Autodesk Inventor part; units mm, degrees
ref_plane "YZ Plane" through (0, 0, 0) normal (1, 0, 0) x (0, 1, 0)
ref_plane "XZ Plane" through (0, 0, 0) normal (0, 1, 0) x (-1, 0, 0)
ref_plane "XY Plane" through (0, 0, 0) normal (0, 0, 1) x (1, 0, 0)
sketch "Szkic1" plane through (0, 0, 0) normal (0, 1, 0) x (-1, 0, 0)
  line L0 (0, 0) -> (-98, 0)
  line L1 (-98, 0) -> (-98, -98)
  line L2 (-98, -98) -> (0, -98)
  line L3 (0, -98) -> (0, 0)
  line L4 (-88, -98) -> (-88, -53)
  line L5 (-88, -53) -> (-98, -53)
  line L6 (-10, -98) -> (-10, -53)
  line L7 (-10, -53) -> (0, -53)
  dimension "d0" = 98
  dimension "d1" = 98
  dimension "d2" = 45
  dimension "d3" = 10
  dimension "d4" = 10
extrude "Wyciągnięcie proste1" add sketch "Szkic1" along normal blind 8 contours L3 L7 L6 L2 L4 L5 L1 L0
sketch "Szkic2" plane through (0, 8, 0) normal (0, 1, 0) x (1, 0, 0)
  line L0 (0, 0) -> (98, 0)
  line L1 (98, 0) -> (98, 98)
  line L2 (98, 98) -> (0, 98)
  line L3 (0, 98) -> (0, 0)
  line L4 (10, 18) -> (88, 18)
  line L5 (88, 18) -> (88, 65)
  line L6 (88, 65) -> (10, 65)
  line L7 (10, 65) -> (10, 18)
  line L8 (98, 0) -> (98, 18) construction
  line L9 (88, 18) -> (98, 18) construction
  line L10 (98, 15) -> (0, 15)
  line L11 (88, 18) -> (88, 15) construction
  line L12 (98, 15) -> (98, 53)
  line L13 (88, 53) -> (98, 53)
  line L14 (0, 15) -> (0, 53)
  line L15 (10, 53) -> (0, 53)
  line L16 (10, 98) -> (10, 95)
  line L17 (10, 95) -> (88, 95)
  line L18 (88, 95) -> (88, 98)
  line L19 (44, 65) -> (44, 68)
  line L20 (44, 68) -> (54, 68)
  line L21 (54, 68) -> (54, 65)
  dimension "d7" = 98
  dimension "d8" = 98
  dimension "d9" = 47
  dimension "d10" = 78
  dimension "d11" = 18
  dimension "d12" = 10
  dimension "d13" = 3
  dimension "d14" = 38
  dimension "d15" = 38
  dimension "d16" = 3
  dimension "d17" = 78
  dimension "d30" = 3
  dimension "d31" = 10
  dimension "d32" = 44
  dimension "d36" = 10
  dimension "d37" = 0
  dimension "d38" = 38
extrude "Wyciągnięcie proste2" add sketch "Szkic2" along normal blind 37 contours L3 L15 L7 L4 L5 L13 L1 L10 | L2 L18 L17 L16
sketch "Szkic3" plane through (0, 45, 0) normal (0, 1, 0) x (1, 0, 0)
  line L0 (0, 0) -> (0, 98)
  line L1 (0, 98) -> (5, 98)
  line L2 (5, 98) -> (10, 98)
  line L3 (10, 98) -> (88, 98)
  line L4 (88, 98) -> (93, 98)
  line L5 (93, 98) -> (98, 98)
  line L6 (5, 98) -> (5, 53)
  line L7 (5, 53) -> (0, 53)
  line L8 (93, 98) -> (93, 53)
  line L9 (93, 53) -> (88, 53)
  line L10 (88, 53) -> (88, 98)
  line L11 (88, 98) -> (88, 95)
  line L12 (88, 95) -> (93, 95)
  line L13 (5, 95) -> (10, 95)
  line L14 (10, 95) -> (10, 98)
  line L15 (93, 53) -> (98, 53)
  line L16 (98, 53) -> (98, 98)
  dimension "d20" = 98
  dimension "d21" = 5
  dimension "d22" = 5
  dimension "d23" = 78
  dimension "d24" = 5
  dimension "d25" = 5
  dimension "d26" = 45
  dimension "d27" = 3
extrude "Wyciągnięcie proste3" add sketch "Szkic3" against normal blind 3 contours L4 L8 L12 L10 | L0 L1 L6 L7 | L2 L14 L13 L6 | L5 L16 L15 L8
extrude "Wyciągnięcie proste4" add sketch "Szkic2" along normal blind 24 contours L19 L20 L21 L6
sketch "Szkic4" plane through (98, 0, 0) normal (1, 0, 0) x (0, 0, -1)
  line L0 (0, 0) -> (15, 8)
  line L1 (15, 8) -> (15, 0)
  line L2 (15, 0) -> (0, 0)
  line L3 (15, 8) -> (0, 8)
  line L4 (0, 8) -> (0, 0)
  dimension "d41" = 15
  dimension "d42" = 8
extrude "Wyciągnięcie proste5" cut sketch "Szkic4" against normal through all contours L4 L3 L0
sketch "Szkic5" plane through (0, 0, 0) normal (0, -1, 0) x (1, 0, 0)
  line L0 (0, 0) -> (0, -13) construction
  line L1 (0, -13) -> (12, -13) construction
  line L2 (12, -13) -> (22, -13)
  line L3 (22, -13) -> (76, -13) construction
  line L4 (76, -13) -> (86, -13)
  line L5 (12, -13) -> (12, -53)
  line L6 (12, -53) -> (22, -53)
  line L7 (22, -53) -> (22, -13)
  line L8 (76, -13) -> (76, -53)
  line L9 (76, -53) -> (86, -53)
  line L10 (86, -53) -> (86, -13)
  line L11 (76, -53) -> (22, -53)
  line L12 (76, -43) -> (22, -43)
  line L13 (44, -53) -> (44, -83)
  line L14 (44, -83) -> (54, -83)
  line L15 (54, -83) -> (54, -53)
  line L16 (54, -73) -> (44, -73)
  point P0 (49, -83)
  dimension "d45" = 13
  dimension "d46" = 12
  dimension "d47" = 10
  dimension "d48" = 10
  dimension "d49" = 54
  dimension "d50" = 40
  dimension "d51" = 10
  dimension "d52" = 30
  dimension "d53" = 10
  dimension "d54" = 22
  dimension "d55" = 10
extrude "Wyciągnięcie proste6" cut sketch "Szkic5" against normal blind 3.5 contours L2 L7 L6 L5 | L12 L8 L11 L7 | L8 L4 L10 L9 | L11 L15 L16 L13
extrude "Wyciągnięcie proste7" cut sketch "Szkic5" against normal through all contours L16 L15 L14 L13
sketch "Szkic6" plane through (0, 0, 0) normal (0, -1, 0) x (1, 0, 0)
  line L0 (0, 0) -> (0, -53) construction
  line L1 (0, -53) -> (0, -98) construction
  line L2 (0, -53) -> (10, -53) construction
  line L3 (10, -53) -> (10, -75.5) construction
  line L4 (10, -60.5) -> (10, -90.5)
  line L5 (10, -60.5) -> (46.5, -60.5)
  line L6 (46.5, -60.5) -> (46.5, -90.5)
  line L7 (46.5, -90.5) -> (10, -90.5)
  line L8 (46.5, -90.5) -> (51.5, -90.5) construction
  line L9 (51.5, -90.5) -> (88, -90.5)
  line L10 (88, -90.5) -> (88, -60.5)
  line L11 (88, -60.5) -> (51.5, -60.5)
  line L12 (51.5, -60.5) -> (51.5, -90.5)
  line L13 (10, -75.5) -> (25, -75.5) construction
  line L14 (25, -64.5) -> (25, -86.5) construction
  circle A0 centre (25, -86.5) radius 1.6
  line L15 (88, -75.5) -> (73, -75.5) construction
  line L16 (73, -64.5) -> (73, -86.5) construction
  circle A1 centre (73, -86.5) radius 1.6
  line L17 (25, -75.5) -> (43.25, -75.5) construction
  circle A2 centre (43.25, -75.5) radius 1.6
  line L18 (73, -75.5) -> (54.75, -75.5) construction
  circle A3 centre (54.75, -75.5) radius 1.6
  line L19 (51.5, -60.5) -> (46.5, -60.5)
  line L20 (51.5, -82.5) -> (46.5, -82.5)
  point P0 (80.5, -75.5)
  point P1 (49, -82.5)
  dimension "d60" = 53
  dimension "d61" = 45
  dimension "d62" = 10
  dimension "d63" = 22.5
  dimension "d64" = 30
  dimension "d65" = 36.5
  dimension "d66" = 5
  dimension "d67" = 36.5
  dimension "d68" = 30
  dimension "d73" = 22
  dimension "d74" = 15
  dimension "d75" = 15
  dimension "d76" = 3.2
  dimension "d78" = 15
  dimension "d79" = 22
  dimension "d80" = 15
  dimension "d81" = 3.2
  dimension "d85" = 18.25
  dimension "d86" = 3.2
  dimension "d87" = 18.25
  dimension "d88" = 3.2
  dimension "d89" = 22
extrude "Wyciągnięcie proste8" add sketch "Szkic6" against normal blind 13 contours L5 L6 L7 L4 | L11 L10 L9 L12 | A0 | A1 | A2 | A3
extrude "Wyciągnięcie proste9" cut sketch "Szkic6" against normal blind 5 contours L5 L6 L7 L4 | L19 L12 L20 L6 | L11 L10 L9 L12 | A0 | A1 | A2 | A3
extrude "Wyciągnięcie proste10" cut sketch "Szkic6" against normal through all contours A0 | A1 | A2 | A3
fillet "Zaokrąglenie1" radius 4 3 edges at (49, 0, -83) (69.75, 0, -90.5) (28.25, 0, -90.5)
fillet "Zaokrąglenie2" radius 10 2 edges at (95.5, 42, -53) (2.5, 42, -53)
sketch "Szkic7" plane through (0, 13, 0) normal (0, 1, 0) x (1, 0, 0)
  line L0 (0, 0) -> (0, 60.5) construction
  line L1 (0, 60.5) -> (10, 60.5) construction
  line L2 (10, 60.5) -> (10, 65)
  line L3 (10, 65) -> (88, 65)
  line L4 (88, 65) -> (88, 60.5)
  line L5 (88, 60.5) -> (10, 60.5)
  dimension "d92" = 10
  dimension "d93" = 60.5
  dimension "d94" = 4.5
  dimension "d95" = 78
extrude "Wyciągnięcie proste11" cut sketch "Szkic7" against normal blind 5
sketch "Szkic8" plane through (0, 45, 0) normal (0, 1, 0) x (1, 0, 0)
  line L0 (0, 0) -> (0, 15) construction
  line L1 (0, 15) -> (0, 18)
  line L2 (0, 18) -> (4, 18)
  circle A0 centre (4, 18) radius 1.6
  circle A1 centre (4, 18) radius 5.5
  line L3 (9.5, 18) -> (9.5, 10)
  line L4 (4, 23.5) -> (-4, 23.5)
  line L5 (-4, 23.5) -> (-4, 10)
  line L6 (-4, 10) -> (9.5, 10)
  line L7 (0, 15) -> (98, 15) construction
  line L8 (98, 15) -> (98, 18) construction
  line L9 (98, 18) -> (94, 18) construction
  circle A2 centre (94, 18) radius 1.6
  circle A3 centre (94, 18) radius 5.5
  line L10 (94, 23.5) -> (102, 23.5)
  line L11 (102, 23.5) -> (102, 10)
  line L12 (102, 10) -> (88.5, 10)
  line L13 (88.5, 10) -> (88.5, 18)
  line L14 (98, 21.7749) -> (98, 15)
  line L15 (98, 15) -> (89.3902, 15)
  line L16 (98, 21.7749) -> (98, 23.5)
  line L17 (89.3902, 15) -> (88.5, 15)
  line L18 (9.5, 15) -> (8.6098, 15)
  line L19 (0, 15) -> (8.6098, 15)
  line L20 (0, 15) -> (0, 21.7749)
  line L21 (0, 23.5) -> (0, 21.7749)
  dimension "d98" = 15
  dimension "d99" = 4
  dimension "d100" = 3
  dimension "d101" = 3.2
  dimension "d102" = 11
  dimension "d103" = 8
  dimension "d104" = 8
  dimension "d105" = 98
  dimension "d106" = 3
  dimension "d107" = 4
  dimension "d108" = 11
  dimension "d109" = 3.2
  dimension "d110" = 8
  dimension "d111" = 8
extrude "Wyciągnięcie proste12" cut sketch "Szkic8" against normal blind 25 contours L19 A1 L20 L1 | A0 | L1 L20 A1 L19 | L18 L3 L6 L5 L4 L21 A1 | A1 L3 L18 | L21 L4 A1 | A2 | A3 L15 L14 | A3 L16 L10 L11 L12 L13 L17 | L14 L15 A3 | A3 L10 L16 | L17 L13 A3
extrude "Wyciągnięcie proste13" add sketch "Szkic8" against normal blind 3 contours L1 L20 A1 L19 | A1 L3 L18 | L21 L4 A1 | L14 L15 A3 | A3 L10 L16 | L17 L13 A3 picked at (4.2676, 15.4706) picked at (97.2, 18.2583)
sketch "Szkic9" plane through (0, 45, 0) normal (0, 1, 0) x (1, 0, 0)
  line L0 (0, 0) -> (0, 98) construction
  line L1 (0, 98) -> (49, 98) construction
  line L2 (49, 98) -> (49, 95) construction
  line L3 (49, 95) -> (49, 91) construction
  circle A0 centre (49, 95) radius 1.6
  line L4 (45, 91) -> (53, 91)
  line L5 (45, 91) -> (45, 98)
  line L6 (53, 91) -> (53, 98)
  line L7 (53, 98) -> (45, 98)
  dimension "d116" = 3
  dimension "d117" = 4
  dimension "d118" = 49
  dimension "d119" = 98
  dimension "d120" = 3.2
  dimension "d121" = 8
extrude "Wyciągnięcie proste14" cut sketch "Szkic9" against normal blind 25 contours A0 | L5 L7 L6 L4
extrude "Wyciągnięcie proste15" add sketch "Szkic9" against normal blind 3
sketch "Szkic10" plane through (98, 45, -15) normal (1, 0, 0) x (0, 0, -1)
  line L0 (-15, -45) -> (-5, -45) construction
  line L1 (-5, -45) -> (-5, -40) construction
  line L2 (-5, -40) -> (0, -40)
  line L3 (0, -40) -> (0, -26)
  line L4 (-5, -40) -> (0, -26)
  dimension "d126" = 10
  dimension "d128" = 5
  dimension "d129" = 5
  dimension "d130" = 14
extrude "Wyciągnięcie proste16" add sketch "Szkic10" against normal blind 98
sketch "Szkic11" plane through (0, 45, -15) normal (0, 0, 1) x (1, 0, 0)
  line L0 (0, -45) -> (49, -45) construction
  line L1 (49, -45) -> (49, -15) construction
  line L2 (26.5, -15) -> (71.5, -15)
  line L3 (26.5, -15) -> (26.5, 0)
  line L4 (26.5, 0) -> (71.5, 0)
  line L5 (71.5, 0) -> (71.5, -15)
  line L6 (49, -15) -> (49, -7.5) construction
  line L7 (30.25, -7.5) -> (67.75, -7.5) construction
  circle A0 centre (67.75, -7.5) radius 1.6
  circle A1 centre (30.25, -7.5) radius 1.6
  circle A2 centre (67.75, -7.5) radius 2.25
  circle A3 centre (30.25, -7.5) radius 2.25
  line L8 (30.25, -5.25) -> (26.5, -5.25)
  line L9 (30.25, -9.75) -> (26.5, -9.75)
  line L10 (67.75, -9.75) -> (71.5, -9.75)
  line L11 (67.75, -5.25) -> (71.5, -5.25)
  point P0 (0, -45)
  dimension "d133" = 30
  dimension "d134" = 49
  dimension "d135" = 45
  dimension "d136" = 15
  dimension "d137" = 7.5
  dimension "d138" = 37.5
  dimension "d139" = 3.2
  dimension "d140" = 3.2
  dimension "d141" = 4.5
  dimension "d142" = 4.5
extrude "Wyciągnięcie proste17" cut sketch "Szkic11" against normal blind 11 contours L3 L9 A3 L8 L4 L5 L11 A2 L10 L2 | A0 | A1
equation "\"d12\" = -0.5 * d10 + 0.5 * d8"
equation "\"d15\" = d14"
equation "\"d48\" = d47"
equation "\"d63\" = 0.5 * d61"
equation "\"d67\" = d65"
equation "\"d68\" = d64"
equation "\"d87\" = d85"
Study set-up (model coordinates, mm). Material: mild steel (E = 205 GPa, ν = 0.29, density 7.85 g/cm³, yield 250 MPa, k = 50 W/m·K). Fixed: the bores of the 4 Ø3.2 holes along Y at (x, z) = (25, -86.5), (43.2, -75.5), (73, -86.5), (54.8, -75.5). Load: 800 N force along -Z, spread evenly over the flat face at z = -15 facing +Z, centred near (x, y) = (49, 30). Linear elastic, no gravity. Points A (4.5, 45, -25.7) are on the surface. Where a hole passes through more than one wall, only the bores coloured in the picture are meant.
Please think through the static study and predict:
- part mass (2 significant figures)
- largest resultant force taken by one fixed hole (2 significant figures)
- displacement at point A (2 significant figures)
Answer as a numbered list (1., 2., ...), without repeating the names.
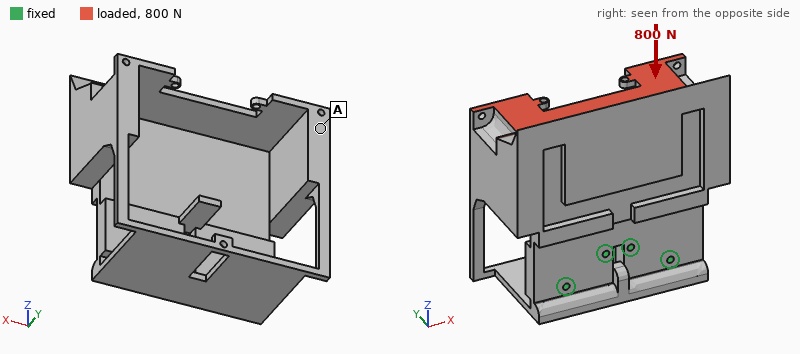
1. 790 g
2. 350 N
3. 0.16 mm
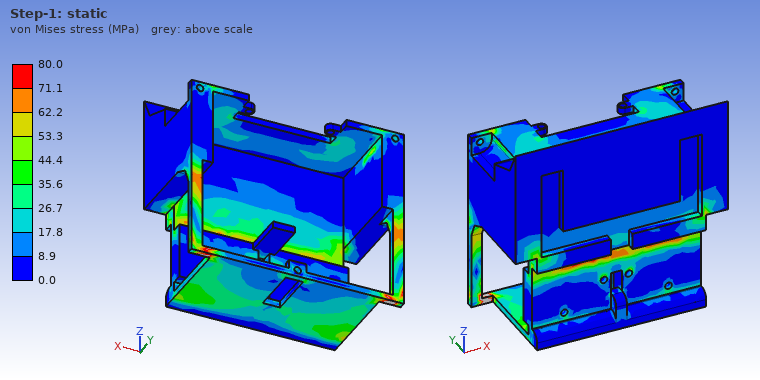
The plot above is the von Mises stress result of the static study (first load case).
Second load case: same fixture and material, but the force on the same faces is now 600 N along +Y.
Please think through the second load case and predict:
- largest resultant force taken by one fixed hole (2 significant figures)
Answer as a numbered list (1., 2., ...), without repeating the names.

1. 590 N
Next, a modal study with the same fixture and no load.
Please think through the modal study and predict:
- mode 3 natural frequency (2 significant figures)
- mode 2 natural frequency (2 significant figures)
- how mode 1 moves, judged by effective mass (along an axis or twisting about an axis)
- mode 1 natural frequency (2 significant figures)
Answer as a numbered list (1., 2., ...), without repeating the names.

1. 2300 Hz
2. 860 Hz
3. along Y
4. 440 Hz
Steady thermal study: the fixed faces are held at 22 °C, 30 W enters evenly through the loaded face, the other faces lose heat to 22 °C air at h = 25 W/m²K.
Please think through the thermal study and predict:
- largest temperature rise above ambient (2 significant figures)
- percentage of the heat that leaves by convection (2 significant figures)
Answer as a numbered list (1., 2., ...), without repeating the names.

1. 61 K
2. 64 %
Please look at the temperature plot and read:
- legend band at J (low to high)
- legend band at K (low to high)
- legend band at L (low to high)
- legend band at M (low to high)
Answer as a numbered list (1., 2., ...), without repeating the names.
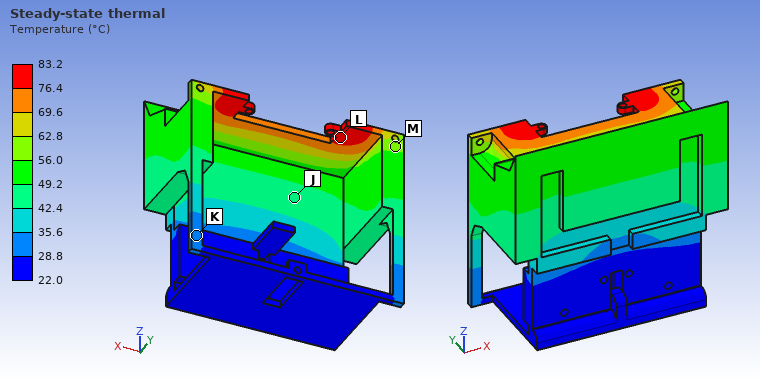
1. 42.4 to 49.2 °C
2. 28.8 to 35.6 °C
3. 76.4 to 83.2 °C
4. 56.0 to 62.8 °C
